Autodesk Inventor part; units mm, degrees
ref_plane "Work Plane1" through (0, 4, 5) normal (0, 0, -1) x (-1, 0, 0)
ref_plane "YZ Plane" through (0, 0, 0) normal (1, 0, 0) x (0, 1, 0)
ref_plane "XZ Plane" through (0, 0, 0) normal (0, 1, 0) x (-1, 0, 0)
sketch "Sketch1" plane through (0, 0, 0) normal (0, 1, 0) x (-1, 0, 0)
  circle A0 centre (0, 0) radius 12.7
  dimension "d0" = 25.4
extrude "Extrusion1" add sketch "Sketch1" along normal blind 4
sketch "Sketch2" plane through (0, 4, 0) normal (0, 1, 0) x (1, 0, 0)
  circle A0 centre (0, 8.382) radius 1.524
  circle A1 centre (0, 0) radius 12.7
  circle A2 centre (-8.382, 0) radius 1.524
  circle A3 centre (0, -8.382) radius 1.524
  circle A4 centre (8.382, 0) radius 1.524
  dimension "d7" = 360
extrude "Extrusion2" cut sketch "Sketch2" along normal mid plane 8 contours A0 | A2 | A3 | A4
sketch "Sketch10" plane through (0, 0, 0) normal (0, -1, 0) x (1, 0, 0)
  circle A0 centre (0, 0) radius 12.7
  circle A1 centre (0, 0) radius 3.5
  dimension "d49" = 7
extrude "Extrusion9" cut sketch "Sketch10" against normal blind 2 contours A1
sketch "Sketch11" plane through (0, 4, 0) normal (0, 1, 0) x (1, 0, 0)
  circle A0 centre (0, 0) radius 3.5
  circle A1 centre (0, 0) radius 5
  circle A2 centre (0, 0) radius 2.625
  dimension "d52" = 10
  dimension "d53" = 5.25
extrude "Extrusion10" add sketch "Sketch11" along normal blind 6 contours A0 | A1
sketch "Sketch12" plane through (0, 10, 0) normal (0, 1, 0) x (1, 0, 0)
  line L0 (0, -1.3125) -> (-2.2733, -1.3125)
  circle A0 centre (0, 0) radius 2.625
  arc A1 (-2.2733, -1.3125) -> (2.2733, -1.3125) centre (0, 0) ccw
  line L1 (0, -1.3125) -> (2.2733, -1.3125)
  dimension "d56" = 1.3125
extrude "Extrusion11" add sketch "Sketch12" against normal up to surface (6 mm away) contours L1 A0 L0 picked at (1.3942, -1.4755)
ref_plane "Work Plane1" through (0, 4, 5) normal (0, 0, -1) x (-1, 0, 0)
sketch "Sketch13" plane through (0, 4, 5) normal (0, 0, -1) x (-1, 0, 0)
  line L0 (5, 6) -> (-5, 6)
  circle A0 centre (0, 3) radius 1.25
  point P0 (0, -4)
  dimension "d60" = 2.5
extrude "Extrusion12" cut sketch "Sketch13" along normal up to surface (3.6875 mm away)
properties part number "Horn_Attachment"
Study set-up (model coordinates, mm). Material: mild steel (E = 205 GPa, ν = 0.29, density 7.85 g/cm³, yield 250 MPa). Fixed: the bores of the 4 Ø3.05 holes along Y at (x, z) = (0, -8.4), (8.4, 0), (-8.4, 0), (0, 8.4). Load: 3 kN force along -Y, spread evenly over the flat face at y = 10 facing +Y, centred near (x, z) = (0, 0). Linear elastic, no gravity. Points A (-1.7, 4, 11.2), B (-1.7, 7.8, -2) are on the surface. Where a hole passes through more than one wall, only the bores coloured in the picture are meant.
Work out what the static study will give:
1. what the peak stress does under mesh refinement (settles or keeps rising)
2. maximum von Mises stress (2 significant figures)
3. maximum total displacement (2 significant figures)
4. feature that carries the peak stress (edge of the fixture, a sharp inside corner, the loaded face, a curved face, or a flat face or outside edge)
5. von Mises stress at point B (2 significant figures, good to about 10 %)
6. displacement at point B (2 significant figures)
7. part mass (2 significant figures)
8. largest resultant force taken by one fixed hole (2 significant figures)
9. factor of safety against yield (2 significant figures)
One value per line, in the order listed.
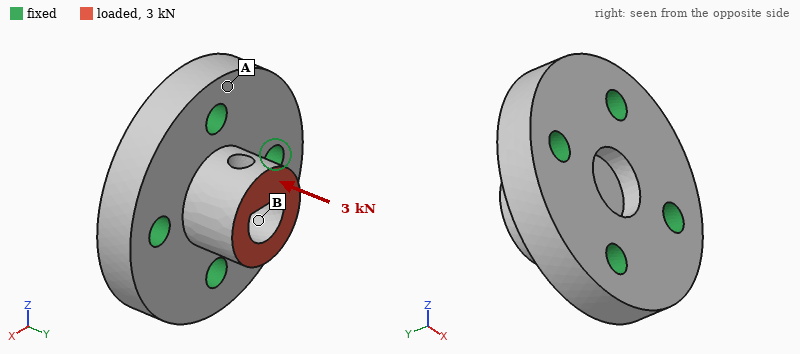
settles
210 MPa
4.9 µm
a curved face
48 MPa
2.7 µm
17 g
820 N
1.2
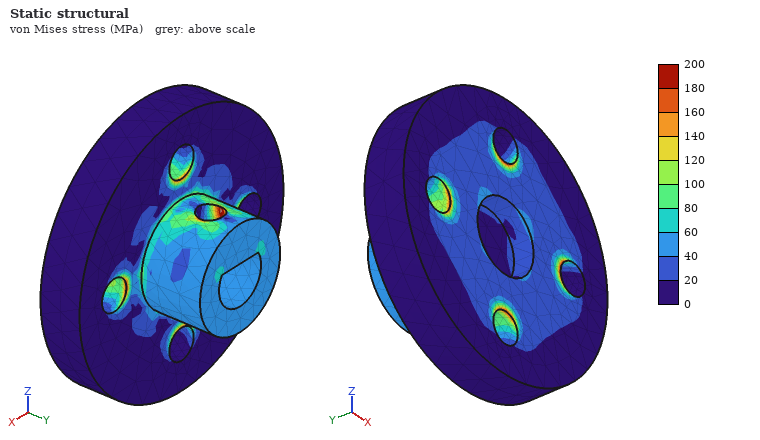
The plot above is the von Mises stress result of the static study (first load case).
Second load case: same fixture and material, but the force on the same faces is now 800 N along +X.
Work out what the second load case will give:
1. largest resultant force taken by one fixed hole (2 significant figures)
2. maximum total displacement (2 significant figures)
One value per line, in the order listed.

510 N
5.1 µm
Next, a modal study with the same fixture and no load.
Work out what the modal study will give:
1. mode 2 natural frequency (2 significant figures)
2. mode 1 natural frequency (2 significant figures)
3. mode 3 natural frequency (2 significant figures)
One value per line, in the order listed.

63 kHz
62 kHz
68 kHz
